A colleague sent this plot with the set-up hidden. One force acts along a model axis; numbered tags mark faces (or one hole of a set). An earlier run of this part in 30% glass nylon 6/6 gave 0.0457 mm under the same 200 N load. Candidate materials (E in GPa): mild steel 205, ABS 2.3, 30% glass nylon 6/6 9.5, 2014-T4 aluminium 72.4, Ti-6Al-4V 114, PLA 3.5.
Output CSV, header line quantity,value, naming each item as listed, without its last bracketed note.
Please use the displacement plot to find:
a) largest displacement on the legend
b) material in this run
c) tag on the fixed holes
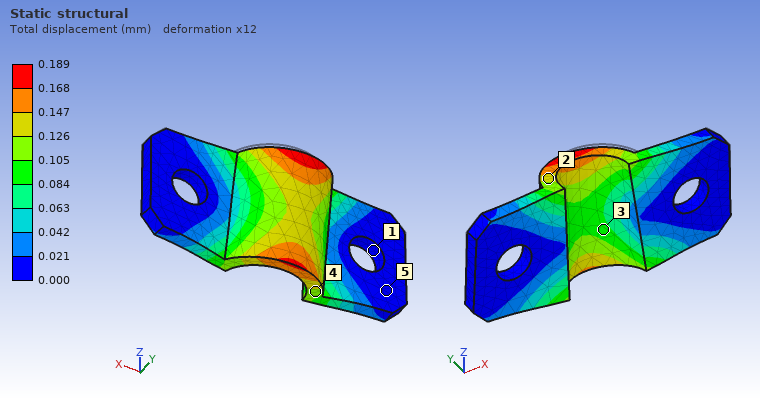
quantity,value
largest displacement on the legend,0.189 mm
material in this run,ABS
tag on the fixed holes,1
